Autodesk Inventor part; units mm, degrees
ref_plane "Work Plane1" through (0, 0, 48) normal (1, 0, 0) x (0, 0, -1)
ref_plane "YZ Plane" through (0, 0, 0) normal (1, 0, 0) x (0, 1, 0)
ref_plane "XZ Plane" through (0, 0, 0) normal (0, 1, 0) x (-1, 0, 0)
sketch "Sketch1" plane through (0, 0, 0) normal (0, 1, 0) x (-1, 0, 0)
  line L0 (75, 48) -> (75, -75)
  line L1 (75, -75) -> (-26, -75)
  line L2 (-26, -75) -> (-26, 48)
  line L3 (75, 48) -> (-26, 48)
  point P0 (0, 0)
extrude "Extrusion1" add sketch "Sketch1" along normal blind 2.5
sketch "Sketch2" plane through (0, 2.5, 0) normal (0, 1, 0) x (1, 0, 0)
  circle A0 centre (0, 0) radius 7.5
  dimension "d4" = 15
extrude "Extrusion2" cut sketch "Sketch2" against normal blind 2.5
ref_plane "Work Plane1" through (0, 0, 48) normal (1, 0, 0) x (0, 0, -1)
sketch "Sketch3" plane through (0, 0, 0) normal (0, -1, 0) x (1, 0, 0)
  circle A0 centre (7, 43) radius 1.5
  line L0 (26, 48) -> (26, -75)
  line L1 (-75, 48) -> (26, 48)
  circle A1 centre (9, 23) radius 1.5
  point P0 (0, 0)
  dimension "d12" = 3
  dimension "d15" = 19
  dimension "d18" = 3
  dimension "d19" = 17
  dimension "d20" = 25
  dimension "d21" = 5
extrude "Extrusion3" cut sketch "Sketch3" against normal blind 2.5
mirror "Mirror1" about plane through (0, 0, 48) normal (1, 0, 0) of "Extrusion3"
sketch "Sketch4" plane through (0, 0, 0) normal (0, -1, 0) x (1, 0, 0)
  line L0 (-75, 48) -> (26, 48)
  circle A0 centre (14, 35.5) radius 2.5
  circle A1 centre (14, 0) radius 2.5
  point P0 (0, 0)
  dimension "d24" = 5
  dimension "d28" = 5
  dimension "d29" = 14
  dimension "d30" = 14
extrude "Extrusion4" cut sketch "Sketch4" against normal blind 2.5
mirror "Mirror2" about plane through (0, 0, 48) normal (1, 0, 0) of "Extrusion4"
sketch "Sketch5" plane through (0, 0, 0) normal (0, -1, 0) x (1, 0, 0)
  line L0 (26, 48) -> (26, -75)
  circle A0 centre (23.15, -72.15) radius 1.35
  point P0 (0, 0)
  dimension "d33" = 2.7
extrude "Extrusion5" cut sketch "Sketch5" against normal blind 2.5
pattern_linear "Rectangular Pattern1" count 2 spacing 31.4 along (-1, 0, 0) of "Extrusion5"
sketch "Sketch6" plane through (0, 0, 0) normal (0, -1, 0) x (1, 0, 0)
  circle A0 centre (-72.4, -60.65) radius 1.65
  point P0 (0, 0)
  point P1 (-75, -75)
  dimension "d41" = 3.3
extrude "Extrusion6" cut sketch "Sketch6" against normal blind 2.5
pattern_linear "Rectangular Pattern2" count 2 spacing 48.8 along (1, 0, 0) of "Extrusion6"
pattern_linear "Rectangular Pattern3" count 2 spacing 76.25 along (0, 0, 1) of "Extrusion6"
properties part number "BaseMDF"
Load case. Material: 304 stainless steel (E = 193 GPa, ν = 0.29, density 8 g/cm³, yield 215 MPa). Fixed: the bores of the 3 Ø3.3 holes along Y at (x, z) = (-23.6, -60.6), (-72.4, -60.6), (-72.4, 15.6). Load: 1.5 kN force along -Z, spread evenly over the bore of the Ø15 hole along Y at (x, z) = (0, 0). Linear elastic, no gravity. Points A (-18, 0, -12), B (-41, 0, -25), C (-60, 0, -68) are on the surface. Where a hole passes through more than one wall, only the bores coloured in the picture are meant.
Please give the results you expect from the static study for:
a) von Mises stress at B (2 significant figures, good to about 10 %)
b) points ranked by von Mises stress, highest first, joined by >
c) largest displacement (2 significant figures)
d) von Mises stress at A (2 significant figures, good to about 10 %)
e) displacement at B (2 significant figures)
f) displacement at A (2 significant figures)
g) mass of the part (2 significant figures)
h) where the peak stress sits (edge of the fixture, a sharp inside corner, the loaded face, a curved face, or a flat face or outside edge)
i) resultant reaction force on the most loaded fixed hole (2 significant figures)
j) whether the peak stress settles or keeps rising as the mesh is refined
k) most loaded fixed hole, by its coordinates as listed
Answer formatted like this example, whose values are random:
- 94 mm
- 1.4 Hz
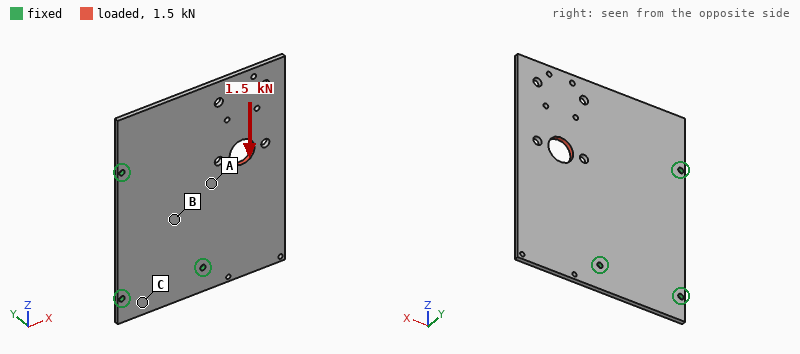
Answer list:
- 6.3 MPa
- A > B > C
- 9.7 µm
- 12 MPa
- 1.8 µm
- 4.2 µm
- 240 g
- edge of the fixture
- 1.3 kN
- keeps rising
- (-23.6, -60.6)
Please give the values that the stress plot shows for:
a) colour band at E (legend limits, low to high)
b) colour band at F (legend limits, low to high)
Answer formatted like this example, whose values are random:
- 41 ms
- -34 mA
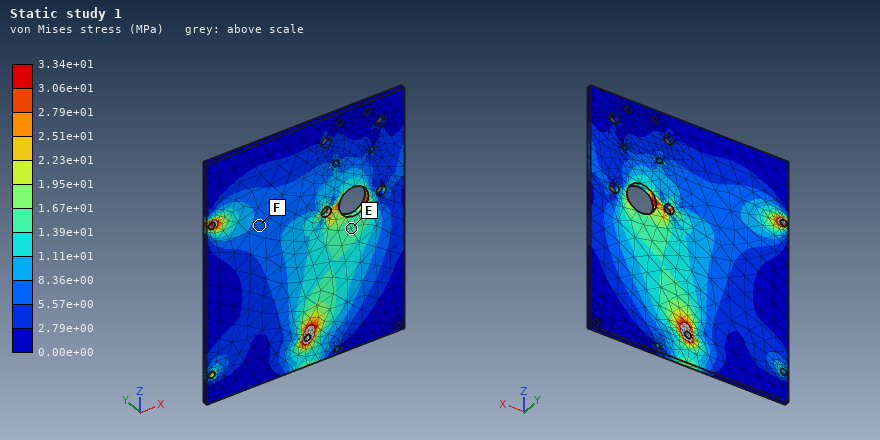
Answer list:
- 1.39e+01 to 1.67e+01 MPa
- 5.57e+00 to 8.36e+00 MPa
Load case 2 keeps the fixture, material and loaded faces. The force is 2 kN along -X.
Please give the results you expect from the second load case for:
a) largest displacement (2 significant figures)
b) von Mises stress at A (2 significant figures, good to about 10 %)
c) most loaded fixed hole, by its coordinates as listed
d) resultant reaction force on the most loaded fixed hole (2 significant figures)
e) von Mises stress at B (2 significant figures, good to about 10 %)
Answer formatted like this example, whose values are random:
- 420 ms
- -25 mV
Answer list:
- 9.3 µm
- 14 MPa
- (-72.4, 15.6)
- 1.4 kN
- 7.3 MPa
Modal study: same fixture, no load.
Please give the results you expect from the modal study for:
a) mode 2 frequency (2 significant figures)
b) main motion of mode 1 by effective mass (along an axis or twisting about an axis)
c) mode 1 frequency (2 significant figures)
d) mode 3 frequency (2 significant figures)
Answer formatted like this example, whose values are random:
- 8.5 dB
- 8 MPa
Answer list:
- 730 Hz
- along Y
- 280 Hz
- 1200 Hz
